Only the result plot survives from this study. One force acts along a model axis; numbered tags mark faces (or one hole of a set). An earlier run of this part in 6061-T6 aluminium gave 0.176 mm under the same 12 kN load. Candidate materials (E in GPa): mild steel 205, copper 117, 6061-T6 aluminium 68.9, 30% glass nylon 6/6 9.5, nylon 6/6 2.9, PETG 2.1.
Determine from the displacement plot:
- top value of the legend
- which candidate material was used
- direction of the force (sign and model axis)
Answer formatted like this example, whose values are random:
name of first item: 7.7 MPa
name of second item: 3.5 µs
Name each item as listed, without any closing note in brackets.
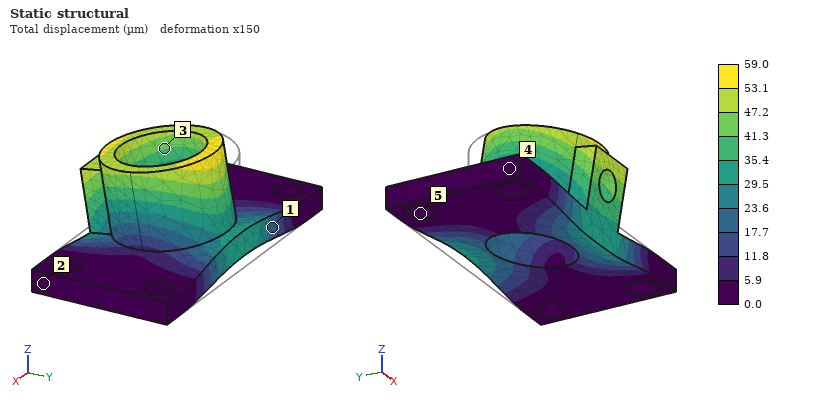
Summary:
top value of the legend: 59.0 µm
which candidate material was used: mild steel
direction of the force: -Y
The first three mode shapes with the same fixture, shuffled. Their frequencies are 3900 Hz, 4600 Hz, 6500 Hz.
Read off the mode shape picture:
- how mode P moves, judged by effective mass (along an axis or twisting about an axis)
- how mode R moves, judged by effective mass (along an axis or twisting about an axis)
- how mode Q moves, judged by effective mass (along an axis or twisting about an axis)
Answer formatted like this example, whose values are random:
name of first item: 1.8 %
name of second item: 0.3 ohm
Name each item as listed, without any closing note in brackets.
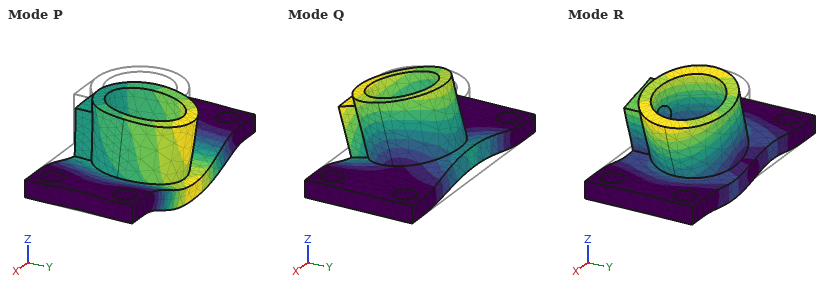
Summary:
how mode P moves, judged by effective mass: along Z
how mode R moves, judged by effective mass: along X
how mode Q moves, judged by effective mass: along Y
